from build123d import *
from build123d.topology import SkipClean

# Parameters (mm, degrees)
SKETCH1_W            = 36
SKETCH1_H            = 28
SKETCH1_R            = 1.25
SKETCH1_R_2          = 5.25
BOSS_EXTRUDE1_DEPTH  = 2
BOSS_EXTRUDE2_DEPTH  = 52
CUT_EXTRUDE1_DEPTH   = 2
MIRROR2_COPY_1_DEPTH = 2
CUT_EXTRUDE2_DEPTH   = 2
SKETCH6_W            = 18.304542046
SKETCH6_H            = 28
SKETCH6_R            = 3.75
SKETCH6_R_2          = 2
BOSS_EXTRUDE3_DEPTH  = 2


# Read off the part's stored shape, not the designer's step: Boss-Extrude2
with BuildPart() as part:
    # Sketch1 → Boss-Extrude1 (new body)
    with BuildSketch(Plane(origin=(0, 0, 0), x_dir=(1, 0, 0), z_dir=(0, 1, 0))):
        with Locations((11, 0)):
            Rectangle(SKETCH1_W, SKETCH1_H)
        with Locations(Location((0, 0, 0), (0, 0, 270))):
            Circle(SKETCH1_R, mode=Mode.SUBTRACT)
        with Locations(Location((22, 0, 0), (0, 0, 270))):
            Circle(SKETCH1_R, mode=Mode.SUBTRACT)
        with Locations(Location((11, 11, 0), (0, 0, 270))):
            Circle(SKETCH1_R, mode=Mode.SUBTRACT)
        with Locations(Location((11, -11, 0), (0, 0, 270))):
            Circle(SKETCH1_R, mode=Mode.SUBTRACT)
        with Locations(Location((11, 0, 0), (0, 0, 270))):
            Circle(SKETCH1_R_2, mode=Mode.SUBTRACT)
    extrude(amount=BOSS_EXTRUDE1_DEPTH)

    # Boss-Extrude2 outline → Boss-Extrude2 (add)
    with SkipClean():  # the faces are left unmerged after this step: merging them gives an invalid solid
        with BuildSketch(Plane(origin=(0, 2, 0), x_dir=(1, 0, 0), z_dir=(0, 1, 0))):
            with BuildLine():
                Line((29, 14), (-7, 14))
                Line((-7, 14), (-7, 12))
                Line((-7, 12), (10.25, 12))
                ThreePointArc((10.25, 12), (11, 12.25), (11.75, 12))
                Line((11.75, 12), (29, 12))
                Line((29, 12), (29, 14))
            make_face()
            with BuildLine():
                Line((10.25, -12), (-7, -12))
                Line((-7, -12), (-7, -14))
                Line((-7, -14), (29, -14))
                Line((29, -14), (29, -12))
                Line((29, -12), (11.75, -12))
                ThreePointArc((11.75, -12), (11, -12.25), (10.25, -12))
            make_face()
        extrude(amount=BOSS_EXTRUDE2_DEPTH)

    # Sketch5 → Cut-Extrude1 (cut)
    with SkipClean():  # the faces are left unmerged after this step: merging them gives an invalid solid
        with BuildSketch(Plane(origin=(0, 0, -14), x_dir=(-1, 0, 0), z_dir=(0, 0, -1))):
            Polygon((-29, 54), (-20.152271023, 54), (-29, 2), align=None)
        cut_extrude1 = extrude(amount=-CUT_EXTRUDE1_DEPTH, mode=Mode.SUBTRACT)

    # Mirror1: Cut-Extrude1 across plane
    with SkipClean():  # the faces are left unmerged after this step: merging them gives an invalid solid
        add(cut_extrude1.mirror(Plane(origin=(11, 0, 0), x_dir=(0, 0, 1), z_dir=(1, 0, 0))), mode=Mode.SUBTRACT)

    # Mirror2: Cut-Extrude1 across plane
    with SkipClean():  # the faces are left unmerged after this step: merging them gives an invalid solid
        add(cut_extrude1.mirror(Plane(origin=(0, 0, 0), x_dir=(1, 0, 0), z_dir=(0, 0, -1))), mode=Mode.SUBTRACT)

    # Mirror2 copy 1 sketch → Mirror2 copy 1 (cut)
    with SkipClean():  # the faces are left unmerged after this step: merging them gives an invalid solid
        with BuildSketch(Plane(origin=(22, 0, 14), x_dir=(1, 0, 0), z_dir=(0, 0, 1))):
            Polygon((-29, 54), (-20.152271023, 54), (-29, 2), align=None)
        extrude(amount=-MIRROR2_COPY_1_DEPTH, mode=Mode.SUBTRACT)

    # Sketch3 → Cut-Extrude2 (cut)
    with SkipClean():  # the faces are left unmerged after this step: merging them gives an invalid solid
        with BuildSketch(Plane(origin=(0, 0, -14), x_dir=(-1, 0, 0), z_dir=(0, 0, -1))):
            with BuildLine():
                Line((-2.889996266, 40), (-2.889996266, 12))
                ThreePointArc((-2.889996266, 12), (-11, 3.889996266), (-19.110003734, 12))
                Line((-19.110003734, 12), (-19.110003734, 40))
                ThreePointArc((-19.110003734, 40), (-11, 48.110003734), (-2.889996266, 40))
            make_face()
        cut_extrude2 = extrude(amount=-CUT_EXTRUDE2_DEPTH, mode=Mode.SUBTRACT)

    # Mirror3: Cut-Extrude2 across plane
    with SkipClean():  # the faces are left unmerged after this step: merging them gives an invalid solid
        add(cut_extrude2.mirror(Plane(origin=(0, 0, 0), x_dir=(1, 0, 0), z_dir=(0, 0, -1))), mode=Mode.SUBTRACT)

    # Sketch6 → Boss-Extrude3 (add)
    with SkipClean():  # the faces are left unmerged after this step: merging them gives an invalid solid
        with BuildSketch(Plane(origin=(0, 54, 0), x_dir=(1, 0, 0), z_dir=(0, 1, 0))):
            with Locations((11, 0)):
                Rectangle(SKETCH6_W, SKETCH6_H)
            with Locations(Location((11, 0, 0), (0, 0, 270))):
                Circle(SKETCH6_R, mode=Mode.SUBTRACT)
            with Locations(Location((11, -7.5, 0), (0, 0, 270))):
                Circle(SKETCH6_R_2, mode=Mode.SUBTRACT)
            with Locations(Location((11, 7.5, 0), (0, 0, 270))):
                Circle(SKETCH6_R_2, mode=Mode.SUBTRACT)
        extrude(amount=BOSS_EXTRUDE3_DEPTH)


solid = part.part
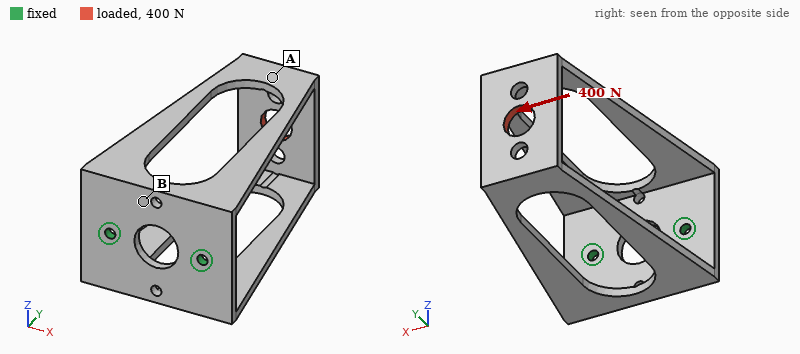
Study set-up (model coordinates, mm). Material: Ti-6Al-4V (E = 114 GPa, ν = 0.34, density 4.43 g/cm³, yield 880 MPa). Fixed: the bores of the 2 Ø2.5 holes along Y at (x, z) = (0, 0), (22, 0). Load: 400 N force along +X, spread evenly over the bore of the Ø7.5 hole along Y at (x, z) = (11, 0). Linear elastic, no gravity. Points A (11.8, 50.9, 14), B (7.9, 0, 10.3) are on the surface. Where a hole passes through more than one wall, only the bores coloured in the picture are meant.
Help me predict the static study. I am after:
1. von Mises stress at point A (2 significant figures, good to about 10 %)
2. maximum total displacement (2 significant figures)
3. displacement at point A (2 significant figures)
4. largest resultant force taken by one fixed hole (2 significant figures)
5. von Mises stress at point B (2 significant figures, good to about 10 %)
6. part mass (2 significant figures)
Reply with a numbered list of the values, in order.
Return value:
1. 67 MPa
2. 0.73 mm
3. 0.67 mm
4. 820 N
5. 150 MPa
6. 25 g
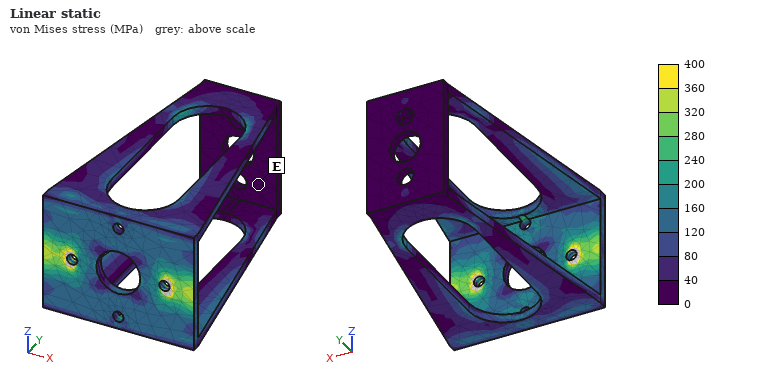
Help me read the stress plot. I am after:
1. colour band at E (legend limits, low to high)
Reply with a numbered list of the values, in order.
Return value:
1. 0 to 40 MPa
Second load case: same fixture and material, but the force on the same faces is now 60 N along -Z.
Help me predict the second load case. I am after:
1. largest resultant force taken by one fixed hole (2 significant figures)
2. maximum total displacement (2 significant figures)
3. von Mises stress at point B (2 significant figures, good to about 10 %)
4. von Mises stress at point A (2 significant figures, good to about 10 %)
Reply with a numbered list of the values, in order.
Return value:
1. 30 N
2. 0.71 mm
3. 34 MPa
4. 29 MPa
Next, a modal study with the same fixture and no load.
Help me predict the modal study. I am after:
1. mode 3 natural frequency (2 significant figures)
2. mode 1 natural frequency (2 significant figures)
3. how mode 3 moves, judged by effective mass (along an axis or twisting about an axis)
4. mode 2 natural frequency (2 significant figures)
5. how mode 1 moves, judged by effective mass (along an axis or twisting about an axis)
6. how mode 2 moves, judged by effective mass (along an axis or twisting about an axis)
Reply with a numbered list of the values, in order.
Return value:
1. 1800 Hz
2. 520 Hz
3. twisting about Y
4. 1300 Hz
5. along Z
6. along X
